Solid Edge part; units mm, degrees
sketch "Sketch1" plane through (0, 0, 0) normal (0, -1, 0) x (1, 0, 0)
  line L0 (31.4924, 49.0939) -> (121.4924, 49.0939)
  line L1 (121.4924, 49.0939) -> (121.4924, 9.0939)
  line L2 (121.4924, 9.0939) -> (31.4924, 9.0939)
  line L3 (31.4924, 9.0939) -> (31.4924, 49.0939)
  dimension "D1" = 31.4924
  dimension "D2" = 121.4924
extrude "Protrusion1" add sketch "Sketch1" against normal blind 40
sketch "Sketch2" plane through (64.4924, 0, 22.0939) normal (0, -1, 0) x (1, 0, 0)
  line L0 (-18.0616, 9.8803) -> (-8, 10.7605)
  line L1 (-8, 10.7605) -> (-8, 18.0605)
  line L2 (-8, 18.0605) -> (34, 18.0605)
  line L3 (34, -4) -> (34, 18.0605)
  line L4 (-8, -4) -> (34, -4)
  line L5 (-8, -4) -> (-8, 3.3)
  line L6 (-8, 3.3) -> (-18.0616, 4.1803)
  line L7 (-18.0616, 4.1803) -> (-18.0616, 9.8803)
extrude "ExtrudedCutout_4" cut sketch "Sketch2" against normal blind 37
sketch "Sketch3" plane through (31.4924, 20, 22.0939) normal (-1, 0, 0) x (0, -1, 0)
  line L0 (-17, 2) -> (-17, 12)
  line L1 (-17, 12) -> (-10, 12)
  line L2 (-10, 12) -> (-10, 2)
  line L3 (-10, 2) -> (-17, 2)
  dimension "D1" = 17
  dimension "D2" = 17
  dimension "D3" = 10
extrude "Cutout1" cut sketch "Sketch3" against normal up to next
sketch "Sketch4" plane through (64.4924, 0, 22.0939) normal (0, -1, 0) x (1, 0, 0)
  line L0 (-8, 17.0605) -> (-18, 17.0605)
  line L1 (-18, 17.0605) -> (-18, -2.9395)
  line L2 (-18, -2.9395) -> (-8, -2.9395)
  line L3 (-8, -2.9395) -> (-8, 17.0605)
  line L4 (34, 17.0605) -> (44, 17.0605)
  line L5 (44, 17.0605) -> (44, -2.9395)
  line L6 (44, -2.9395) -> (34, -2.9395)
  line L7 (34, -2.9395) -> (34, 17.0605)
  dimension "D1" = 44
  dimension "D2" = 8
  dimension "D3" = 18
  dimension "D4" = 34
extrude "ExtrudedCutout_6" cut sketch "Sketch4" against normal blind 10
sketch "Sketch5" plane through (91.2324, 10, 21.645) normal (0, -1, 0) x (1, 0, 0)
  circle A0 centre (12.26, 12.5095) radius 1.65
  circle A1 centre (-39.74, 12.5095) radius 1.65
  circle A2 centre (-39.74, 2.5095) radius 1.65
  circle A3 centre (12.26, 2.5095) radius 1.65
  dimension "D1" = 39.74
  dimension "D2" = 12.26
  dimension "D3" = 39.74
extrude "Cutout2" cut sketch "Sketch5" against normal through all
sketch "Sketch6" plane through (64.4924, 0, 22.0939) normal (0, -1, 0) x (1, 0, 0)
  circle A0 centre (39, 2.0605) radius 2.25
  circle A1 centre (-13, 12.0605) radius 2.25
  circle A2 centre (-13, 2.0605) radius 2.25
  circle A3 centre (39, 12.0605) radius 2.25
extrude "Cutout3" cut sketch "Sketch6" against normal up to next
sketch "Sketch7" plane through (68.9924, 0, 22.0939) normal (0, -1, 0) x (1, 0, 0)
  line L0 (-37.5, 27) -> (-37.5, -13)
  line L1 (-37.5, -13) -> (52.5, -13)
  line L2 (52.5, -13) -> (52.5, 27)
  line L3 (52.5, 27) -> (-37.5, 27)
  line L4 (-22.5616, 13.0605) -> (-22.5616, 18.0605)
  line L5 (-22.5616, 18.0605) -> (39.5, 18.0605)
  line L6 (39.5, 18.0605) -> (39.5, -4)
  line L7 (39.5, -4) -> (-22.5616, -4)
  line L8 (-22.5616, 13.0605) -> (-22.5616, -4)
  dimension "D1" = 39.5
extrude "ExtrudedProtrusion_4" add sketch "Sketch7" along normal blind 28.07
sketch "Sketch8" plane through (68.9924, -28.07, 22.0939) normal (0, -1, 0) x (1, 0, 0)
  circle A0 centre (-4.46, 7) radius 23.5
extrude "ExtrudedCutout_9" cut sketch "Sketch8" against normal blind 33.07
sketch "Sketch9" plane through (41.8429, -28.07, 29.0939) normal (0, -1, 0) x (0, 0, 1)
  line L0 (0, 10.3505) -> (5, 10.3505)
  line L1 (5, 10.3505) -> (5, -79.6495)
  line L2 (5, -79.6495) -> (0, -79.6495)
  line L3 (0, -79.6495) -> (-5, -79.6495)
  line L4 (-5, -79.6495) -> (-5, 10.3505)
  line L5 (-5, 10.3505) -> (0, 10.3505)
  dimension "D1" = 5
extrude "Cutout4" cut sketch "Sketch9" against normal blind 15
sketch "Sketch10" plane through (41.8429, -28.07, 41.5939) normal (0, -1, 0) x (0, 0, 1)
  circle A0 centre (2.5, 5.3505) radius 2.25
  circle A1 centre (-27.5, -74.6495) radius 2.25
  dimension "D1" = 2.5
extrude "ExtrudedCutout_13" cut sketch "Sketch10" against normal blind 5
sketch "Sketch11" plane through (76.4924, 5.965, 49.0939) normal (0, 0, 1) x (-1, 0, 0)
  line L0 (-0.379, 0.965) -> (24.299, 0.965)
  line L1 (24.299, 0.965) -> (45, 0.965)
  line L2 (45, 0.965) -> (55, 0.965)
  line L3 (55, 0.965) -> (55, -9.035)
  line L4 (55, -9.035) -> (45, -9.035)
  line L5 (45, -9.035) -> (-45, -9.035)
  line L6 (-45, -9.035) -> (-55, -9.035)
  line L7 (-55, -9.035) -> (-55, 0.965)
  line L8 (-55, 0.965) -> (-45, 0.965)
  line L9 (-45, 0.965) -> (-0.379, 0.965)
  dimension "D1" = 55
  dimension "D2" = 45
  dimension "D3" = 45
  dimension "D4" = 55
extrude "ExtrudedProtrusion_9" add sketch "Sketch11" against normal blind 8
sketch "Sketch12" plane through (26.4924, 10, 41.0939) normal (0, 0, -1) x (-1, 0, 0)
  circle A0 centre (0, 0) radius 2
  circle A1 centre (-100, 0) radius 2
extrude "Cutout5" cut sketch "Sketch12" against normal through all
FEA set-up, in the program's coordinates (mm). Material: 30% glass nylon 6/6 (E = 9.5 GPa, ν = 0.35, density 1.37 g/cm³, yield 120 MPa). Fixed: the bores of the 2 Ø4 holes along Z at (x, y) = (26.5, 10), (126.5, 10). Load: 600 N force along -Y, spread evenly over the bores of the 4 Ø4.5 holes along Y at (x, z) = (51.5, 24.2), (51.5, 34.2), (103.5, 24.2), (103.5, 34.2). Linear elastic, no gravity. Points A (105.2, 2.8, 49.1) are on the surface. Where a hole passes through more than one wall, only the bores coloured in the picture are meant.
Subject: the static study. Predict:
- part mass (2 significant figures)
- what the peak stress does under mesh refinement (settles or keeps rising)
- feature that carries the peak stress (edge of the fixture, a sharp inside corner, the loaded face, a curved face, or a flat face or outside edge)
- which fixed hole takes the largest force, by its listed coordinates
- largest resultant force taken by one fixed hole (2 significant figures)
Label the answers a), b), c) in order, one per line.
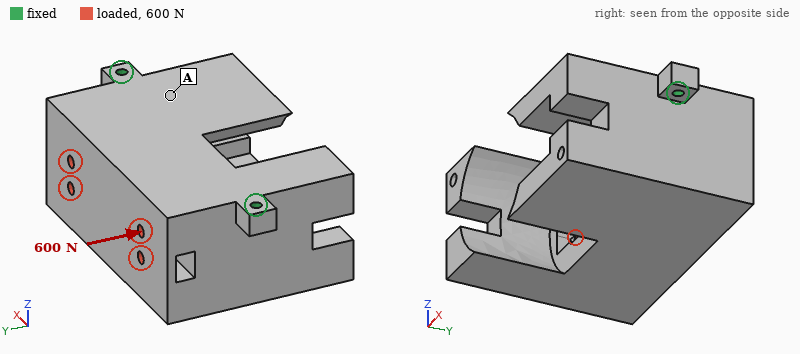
a) 190 g
b) keeps rising
c) edge of the fixture
d) (126.5, 10)
e) 350 N
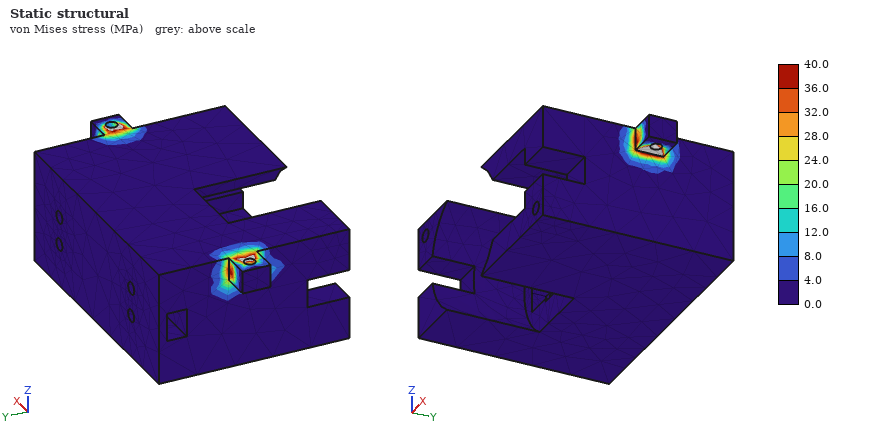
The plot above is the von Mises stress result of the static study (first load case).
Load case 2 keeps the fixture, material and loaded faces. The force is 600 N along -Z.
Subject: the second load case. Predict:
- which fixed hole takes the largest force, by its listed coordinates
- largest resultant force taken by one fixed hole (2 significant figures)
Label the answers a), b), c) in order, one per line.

a) (126.5, 10)
b) 350 N
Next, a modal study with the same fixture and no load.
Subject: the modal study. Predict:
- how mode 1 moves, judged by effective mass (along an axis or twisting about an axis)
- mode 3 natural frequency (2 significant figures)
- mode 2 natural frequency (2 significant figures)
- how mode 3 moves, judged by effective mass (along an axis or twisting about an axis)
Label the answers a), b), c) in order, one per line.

a) along Y
b) 2300 Hz
c) 1600 Hz
d) along Z
